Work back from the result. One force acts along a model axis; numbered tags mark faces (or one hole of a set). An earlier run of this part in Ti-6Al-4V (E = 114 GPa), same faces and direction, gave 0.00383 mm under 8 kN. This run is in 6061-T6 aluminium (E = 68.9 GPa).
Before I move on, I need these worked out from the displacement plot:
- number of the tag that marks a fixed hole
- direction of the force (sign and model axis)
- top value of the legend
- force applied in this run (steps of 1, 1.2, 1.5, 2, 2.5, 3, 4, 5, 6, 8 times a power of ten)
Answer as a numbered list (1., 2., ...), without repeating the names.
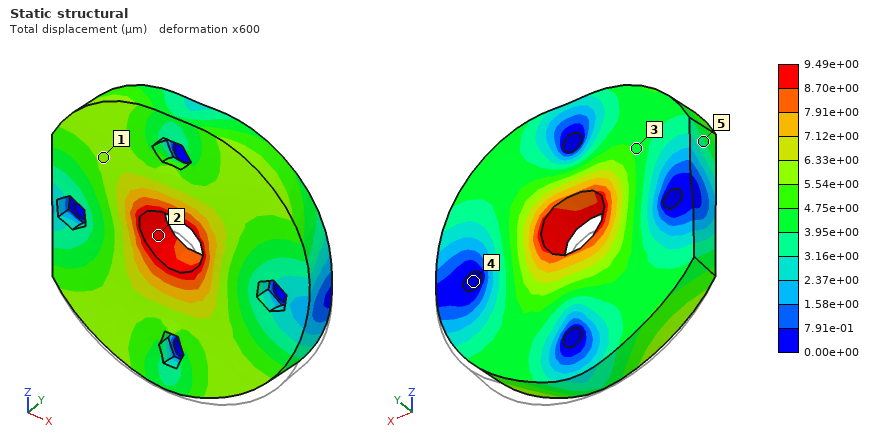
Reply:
1. 4
2. +Z
3. 9.49e+00 µm
4. 12 kN
